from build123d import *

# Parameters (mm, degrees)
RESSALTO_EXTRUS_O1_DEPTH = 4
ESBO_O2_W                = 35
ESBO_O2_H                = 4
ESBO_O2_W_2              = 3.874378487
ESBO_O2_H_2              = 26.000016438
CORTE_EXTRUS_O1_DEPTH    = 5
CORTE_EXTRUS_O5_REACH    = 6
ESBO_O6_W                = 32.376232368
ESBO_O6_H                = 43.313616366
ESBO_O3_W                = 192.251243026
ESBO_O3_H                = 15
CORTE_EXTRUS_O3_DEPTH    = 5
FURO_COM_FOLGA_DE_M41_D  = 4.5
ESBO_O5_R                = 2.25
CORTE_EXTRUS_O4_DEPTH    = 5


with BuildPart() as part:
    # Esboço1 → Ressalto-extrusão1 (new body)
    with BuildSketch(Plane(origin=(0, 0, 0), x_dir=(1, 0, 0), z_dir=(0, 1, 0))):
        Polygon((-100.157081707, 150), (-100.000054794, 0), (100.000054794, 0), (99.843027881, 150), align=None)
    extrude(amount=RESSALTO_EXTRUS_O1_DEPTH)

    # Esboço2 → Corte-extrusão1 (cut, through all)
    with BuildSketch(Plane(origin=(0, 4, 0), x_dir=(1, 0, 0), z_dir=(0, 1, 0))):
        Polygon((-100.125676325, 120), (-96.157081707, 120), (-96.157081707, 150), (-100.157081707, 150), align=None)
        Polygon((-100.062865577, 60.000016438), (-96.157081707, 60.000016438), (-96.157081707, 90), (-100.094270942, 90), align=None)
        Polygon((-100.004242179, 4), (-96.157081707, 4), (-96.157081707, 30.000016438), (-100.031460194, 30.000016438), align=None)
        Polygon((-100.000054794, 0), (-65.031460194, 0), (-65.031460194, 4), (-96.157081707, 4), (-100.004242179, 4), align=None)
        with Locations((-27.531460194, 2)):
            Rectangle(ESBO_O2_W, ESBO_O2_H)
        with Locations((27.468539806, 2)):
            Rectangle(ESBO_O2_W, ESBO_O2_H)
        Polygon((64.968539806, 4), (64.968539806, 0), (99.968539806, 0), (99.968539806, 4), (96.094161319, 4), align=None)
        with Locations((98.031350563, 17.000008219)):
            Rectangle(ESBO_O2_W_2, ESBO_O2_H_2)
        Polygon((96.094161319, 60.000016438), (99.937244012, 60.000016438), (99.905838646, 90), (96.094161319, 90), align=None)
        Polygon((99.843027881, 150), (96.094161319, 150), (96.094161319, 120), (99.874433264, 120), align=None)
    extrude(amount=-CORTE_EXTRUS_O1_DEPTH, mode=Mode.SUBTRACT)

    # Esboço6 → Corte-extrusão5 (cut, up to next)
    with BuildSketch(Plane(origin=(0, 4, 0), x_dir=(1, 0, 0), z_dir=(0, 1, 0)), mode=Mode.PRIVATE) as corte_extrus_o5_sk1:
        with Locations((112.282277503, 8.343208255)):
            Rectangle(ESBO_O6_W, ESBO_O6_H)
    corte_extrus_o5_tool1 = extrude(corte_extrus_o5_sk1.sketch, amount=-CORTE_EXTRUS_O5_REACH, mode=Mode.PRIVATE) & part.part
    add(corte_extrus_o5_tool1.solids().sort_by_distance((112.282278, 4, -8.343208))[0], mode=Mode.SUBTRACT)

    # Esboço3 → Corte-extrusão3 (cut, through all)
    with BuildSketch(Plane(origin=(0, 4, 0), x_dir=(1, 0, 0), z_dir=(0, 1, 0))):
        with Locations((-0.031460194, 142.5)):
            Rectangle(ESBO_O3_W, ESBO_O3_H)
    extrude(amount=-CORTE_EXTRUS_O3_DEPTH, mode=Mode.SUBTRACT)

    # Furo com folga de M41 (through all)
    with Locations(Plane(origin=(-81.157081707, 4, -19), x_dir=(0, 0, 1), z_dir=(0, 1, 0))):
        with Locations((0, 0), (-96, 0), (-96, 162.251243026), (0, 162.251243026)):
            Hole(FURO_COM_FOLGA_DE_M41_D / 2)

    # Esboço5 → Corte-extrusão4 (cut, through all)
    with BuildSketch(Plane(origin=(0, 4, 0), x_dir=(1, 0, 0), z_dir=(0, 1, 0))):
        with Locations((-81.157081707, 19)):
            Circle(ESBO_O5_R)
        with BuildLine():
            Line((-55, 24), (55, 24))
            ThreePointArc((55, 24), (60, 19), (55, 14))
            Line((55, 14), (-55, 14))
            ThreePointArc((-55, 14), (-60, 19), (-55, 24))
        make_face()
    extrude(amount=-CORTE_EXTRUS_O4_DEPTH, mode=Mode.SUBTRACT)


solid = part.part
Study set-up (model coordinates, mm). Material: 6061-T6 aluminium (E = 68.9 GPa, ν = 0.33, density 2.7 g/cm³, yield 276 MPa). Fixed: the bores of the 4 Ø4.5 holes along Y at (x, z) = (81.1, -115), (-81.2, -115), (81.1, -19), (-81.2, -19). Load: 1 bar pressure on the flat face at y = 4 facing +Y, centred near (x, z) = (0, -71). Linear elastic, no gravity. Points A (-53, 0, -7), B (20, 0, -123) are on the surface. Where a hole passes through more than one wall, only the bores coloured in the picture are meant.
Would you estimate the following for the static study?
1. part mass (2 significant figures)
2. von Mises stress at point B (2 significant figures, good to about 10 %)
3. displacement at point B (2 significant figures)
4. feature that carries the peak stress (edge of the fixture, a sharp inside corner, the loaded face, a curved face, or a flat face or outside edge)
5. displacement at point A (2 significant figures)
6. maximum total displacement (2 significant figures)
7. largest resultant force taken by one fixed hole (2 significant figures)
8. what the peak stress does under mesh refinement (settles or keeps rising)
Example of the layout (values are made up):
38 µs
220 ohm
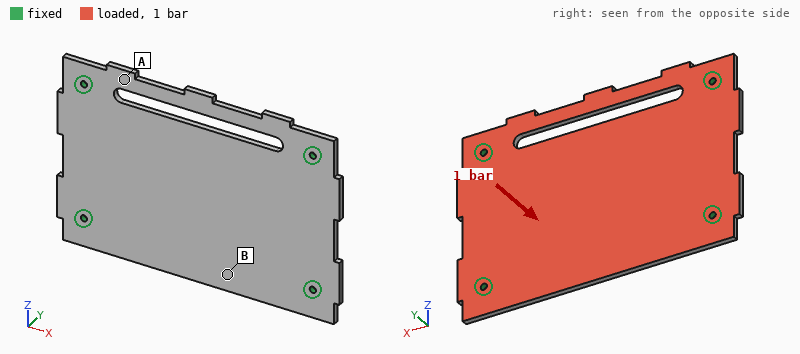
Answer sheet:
270 g
41 MPa
0.57 mm
edge of the fixture
0.18 mm
0.71 mm
670 N
keeps rising
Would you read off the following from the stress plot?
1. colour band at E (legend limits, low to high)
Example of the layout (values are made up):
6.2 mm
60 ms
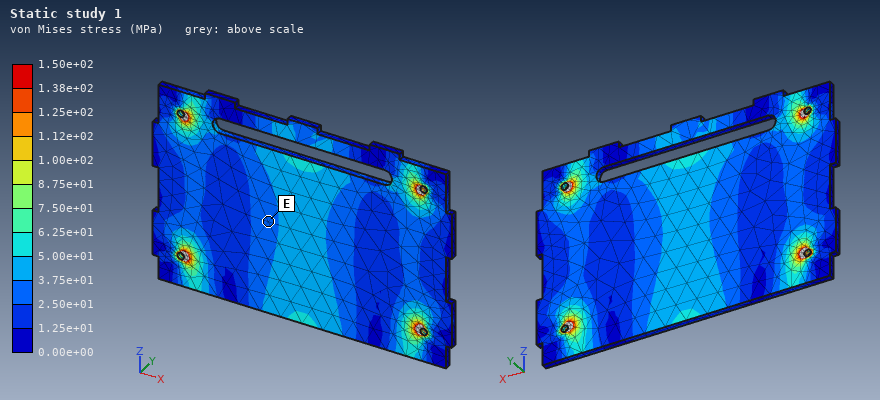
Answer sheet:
2.50e+01 to 3.75e+01 MPa
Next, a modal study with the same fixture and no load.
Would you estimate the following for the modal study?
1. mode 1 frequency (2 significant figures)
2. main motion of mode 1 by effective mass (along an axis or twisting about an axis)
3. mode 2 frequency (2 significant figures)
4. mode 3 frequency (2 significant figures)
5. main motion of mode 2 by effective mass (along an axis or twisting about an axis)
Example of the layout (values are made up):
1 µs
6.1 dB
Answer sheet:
670 Hz
along Y
940 Hz
1100 Hz
twisting about X
